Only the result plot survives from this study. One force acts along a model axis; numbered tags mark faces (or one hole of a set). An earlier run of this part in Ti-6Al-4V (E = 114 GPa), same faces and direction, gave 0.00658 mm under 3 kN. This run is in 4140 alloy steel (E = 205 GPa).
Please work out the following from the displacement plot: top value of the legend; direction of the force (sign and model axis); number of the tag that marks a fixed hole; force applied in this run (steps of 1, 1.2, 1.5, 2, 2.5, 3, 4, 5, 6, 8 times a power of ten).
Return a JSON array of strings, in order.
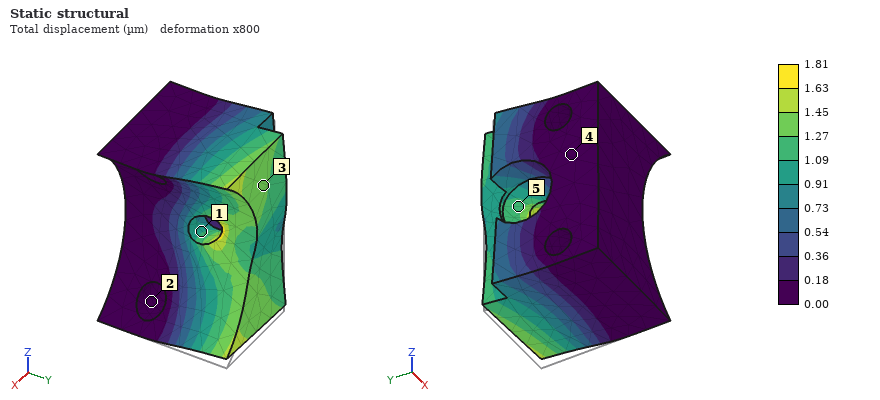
["1.81 µm", "+Z", "2", "1.5 kN"]
